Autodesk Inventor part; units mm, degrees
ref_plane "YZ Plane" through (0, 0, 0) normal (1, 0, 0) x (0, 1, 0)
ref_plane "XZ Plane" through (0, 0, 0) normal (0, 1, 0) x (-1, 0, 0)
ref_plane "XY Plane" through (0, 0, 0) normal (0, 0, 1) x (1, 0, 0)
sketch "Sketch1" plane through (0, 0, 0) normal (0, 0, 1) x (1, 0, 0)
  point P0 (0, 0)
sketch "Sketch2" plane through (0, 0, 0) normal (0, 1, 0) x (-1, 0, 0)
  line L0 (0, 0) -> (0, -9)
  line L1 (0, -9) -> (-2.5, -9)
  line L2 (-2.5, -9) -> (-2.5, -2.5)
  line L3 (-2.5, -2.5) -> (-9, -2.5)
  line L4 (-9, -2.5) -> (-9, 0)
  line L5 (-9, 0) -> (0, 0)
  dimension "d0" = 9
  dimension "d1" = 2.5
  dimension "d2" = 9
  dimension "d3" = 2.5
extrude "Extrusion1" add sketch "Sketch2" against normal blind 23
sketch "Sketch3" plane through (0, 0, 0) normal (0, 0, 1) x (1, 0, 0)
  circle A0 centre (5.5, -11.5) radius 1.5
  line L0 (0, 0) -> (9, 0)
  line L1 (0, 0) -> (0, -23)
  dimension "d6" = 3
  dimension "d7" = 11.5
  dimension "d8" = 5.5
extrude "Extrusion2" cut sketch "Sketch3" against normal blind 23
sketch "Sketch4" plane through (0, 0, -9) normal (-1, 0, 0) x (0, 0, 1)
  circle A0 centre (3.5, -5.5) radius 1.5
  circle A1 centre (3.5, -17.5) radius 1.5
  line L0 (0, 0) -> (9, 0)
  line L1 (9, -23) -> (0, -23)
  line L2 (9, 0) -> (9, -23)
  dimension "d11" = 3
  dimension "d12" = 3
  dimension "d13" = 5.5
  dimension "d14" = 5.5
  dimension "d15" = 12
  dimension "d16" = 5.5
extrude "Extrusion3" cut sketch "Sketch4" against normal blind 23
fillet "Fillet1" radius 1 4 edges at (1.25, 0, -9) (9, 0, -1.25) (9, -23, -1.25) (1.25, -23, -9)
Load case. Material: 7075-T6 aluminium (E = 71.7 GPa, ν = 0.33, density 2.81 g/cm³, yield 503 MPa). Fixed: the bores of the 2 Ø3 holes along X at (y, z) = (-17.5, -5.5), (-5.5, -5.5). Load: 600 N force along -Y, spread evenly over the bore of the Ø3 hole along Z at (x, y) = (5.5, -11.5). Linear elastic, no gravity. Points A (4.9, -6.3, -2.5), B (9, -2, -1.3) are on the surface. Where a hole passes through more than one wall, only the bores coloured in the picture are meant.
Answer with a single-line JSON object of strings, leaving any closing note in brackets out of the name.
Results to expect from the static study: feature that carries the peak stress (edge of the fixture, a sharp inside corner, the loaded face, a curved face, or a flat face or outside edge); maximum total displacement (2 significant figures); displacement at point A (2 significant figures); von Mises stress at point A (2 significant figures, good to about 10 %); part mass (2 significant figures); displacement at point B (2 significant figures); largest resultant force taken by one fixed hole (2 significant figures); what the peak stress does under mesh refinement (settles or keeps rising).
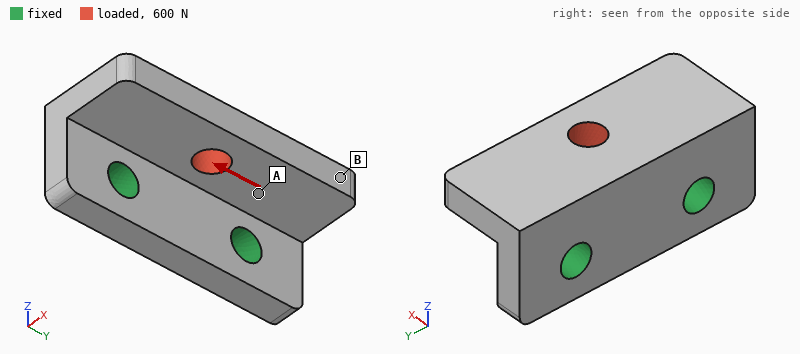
{"feature that carries the peak stress": "edge of the fixture", "maximum total displacement": "12 µm", "displacement at point A": "5.5 µm", "von Mises stress at point A": "28 MPa", "part mass": "2.3 g", "displacement at point B": "11 µm", "largest resultant force taken by one fixed hole": "380 N", "what the peak stress does under mesh refinement": "keeps rising"}
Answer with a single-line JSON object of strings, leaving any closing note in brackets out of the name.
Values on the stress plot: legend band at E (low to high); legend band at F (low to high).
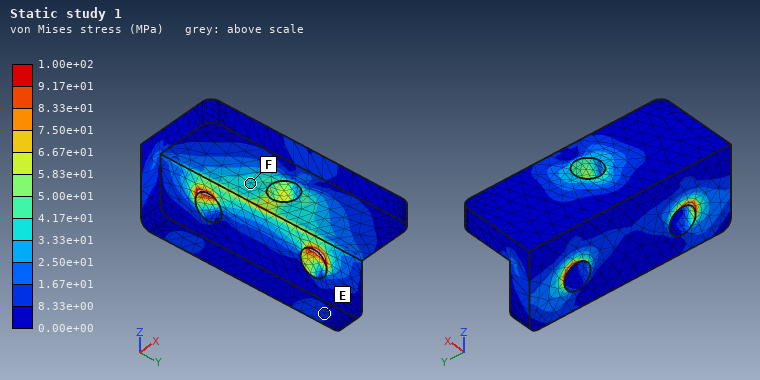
{"legend band at E": "8.33e+00 to 1.67e+01 MPa", "legend band at F": "3.33e+01 to 4.17e+01 MPa"}
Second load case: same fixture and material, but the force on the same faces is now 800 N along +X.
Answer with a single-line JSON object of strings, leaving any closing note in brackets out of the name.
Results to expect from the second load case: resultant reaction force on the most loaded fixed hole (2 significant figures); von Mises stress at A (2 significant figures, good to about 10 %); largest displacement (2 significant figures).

{"resultant reaction force on the most loaded fixed hole": "410 N", "von Mises stress at A": "22 MPa", "largest displacement": "31 µm"}
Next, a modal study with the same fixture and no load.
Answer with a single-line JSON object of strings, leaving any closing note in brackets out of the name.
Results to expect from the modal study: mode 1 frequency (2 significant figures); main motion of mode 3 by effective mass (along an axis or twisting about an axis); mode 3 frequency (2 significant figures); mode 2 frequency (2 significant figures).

{"mode 1 frequency": "20 kHz", "main motion of mode 3 by effective mass": "along Y", "mode 3 frequency": "42 kHz", "mode 2 frequency": "26 kHz"}
